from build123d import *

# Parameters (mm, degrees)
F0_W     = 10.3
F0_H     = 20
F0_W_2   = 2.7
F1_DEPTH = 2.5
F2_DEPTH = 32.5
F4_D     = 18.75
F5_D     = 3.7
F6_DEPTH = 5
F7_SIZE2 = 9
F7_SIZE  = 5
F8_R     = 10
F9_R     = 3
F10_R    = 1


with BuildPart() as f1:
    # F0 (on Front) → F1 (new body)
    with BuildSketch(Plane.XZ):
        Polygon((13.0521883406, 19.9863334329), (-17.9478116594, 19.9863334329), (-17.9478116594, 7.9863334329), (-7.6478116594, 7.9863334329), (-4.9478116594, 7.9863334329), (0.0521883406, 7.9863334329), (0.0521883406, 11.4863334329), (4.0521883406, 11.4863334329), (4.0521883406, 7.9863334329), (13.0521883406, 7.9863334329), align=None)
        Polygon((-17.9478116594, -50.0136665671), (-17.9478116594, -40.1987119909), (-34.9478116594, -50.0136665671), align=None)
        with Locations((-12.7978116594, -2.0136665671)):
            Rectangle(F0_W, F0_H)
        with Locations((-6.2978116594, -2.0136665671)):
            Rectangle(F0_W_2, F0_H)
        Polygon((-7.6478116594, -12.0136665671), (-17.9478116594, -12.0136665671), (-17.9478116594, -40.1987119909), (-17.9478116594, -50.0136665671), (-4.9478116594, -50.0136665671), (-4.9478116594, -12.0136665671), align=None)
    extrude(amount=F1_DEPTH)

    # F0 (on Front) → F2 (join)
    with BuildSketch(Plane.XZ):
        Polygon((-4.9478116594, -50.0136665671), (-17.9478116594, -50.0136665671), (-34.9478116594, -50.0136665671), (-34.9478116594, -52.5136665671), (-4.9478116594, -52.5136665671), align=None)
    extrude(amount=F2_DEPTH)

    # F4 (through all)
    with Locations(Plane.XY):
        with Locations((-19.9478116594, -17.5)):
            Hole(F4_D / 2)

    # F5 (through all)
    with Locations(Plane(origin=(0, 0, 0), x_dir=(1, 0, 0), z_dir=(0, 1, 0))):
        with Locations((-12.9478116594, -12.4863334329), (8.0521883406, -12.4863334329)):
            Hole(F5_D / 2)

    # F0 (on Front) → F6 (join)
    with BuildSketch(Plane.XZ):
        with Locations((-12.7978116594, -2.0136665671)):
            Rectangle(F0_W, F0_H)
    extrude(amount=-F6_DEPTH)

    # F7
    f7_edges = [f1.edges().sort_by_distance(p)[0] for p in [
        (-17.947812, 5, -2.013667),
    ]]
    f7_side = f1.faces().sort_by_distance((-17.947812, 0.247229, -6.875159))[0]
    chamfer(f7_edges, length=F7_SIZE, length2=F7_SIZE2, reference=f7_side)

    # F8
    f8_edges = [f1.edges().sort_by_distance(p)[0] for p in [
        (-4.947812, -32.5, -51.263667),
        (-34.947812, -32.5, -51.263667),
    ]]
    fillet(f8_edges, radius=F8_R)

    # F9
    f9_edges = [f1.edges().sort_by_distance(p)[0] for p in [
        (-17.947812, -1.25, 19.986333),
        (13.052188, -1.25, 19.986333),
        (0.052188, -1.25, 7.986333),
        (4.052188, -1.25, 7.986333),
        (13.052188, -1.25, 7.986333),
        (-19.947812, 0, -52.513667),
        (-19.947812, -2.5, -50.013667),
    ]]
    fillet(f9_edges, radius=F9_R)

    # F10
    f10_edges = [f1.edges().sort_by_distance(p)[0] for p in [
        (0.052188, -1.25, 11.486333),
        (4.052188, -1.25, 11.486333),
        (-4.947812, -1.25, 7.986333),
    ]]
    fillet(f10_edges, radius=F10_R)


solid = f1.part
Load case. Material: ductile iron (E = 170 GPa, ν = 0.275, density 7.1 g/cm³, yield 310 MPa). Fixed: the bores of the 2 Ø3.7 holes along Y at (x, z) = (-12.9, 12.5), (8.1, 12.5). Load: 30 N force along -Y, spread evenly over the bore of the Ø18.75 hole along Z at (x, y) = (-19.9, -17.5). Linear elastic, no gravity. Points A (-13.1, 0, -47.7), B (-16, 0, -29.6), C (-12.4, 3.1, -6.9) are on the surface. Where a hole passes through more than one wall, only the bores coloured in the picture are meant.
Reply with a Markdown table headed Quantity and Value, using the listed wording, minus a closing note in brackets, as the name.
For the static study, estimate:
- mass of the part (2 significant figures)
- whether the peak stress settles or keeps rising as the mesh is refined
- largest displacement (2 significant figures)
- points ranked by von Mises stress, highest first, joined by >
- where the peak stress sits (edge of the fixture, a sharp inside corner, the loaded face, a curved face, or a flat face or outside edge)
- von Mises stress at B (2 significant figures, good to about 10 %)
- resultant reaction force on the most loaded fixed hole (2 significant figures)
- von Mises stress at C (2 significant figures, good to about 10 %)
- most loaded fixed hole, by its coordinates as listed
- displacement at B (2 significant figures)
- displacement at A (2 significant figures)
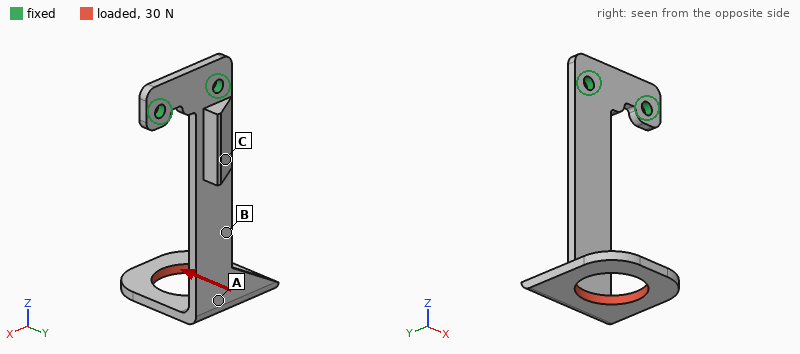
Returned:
| Quantity | Value |
|---|---|
| mass of the part | 36 g |
| whether the peak stress settles or keeps rising as the mesh is refined | keeps rising |
| largest displacement | 0.64 mm |
| points ranked by von Mises stress, highest first, joined by > | B > C > A |
| where the peak stress sits | edge of the fixture |
| von Mises stress at B | 52 MPa |
| resultant reaction force on the most loaded fixed hole | 44 N |
| von Mises stress at C | 27 MPa |
| most loaded fixed hole, by its coordinates as listed | (-12.9, 12.5) |
| displacement at B | 0.21 mm |
| displacement at A | 0.42 mm |
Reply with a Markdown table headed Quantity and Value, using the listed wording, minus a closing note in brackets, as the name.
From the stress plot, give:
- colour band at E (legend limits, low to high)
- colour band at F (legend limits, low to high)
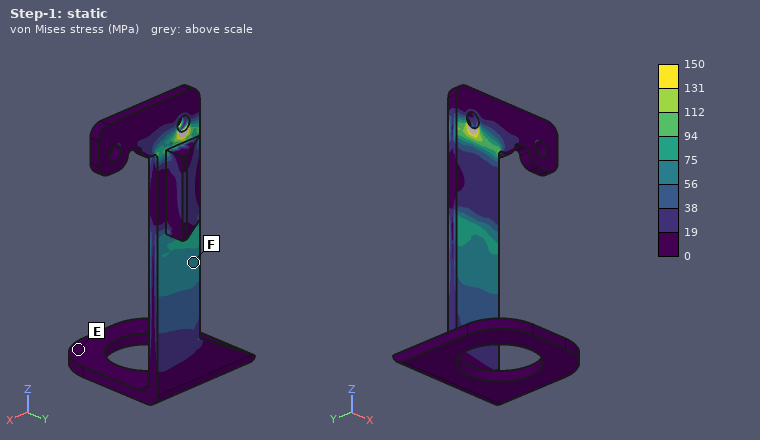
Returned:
| Quantity | Value |
|---|---|
| colour band at E | 0 to 19 MPa |
| colour band at F | 56 to 75 MPa |
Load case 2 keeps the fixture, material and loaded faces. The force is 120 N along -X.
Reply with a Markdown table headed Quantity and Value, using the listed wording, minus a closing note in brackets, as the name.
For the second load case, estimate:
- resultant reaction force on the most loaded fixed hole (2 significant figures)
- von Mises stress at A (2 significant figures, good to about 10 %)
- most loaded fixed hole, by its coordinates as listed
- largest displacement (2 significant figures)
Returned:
| Quantity | Value |
|---|---|
| resultant reaction force on the most loaded fixed hole | 330 N |
| von Mises stress at A | 59 MPa |
| most loaded fixed hole, by its coordinates as listed | (-12.9, 12.5) |
| largest displacement | 0.81 mm |
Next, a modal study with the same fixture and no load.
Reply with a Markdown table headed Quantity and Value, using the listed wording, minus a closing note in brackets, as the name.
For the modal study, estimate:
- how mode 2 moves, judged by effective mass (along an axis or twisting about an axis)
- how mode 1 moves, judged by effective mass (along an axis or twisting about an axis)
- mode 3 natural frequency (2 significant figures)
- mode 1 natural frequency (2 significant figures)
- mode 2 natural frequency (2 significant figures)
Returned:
| Quantity | Value |
|---|---|
| how mode 2 moves, judged by effective mass | along X |
| how mode 1 moves, judged by effective mass | along Y |
| mode 3 natural frequency | 1100 Hz |
| mode 1 natural frequency | 300 Hz |
| mode 2 natural frequency | 680 Hz |
